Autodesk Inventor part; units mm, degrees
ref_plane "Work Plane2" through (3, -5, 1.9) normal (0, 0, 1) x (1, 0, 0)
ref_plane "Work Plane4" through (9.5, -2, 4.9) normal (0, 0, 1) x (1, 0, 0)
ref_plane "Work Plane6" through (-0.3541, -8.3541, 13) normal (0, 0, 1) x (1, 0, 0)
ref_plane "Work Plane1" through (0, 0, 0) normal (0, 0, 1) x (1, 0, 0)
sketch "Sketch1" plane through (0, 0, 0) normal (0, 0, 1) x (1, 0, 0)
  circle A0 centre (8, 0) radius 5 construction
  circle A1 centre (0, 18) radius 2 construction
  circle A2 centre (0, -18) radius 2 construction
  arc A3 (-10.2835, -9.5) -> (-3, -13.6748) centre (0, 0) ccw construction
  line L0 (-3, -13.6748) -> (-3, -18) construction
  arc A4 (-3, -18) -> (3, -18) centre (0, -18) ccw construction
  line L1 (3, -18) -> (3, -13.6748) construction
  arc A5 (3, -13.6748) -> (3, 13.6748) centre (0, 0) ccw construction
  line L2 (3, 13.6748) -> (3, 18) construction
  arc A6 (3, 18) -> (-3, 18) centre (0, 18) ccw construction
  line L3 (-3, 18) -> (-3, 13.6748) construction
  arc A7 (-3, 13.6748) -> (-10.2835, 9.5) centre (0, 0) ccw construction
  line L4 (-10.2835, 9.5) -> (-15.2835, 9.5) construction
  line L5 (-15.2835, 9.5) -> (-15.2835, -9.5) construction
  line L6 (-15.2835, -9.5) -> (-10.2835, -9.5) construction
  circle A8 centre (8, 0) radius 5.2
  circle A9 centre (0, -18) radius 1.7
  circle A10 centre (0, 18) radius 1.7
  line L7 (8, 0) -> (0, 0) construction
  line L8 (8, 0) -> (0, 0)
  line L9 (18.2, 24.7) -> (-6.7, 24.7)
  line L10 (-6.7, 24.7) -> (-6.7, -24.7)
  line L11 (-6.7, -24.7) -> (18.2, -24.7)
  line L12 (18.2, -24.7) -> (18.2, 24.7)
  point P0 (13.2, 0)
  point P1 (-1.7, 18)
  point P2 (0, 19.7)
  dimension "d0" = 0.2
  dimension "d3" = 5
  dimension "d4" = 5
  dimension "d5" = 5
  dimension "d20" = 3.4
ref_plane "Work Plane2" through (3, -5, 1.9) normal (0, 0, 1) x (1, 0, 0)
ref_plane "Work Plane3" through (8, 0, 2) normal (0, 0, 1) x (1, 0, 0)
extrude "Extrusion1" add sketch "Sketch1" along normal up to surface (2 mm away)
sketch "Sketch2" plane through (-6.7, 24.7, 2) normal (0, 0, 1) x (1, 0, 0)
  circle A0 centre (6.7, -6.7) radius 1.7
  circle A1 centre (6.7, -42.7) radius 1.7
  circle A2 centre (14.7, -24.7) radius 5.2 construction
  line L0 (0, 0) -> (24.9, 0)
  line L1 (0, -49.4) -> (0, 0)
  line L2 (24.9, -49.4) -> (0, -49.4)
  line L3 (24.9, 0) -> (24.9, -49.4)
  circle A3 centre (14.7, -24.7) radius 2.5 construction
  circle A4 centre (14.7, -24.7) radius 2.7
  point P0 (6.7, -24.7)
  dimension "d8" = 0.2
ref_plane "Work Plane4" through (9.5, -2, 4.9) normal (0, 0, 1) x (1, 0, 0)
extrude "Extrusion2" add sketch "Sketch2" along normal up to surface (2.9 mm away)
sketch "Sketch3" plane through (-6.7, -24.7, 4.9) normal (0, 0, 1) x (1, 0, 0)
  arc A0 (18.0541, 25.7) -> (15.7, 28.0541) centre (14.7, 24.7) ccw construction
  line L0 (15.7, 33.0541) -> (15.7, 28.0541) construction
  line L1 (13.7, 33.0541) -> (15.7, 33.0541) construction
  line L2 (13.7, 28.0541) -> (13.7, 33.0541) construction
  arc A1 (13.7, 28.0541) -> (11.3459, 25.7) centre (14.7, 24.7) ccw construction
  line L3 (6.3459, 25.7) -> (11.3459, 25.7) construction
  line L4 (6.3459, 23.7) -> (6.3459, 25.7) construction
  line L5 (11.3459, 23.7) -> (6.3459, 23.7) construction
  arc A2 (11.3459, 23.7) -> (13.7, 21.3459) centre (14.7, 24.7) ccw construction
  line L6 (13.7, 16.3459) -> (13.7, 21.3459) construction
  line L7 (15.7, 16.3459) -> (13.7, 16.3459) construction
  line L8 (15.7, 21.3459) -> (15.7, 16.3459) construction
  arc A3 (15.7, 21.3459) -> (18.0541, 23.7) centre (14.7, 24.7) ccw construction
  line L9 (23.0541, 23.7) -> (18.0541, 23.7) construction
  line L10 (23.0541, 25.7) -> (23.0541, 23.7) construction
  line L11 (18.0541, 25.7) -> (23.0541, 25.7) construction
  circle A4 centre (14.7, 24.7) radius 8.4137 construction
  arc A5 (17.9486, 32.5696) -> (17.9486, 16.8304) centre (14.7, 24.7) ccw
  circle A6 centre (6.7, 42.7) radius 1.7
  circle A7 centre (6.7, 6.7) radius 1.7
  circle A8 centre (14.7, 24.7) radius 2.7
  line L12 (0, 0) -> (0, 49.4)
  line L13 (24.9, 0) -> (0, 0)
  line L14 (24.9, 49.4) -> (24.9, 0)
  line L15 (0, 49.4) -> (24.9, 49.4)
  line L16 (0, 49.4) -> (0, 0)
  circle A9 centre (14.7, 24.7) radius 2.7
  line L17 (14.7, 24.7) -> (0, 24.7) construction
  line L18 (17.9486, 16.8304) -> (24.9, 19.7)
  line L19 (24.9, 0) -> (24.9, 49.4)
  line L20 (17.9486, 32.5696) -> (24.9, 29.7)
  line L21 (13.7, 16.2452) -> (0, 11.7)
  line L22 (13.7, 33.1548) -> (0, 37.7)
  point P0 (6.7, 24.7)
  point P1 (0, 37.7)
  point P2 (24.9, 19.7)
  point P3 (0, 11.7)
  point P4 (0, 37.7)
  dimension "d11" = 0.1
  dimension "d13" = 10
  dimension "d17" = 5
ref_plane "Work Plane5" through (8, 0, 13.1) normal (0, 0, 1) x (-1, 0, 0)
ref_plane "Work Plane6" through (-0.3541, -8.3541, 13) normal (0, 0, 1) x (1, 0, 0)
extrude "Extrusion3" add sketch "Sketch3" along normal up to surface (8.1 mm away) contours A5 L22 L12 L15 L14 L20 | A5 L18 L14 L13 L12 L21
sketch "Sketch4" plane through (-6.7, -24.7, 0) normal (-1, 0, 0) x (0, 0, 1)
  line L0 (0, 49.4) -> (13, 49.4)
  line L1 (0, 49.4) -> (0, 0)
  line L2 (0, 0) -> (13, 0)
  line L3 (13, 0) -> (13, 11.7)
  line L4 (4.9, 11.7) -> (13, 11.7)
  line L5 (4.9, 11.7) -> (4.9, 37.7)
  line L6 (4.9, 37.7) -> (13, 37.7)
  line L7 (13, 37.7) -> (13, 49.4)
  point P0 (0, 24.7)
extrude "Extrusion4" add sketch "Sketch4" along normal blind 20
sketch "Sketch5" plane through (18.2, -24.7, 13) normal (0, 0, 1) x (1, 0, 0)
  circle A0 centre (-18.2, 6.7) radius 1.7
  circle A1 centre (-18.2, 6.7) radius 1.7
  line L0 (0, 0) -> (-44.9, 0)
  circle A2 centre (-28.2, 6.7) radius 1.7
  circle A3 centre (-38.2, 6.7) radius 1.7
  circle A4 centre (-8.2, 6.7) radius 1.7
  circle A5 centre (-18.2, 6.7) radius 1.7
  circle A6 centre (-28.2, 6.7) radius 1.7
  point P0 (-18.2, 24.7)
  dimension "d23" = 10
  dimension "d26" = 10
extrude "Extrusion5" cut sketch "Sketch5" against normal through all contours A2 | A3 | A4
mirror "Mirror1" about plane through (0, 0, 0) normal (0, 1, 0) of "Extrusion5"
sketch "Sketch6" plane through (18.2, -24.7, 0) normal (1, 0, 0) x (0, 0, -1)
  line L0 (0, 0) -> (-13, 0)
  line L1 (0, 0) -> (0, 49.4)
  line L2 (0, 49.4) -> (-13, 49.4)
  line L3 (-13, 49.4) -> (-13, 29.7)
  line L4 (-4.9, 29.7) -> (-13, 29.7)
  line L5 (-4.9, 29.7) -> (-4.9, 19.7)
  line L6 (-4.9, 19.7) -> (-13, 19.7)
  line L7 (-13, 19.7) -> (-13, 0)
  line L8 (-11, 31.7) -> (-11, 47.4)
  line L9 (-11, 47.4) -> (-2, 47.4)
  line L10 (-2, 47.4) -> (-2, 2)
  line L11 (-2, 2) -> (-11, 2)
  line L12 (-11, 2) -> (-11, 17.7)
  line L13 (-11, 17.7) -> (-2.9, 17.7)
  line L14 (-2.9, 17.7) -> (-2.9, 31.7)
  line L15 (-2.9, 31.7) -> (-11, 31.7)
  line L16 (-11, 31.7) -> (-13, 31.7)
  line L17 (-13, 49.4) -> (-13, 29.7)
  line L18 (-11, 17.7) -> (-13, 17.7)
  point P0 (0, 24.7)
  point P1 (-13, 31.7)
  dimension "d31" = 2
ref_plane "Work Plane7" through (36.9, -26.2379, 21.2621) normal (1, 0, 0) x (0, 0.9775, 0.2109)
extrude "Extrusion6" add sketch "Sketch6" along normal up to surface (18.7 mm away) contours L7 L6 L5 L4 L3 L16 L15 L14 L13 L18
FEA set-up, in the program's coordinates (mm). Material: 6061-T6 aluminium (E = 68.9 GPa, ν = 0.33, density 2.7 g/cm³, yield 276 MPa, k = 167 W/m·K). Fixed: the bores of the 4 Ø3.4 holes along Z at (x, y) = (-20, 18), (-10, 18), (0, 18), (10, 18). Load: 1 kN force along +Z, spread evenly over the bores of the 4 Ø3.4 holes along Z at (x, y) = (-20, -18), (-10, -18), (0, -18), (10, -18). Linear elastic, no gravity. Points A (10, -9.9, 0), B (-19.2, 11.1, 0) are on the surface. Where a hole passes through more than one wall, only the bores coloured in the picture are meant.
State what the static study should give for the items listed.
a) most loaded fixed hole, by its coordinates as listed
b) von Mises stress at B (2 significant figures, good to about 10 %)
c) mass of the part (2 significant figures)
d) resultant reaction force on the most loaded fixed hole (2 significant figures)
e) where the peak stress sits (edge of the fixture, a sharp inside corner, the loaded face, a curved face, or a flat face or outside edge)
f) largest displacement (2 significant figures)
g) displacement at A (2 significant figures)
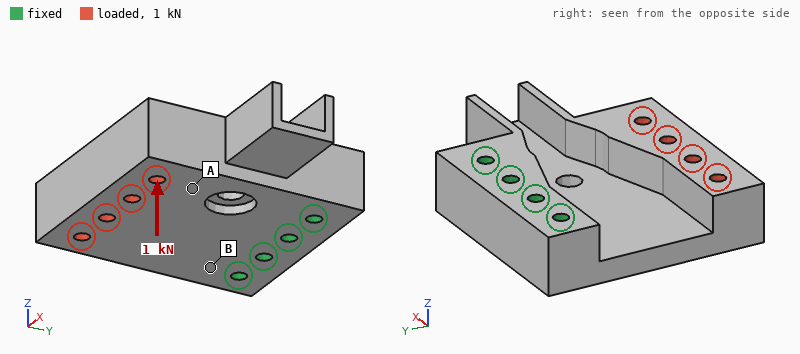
(0, 18)
130 MPa
56 g
410 N
a curved face
0.49 mm
0.19 mm
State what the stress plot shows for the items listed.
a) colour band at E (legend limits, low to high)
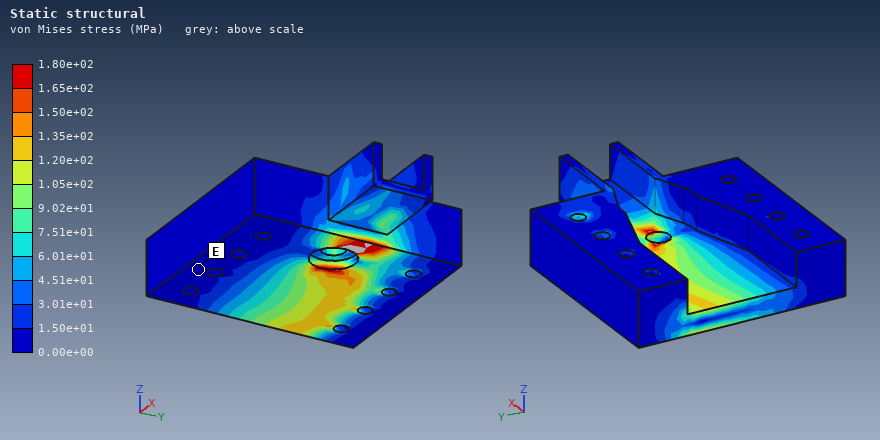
0.00e+00 to 1.50e+01 MPa
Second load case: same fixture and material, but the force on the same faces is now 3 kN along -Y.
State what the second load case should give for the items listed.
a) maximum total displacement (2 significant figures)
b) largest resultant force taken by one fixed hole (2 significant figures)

0.27 mm
1.0 kN
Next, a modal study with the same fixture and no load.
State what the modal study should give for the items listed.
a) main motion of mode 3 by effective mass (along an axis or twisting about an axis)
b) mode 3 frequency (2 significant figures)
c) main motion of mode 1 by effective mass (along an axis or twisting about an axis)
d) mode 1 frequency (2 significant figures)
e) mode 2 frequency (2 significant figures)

along X
8200 Hz
along Z
1800 Hz
4600 Hz
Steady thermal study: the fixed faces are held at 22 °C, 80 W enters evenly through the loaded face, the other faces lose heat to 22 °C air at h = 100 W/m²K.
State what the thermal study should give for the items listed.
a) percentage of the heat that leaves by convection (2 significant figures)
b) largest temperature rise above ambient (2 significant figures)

27 %
56 K
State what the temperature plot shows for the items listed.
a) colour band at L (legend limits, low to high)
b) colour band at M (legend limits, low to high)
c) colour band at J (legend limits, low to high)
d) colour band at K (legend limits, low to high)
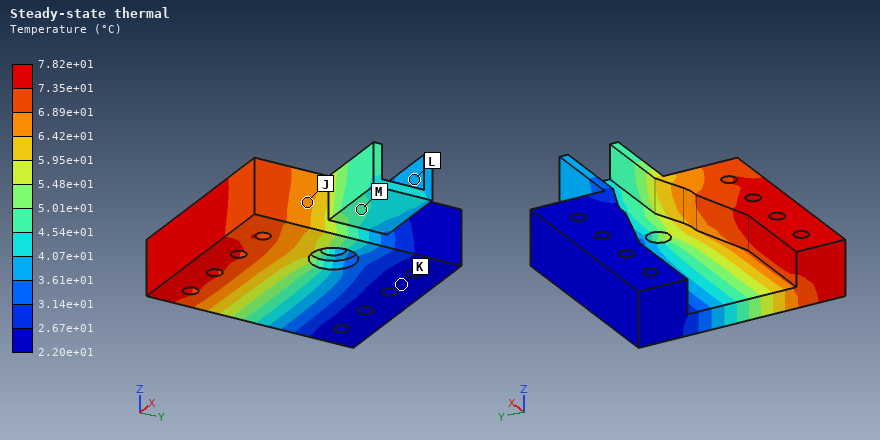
3.61e+01 to 4.07e+01 °C
4.54e+01 to 5.01e+01 °C
6.42e+01 to 6.89e+01 °C
2.20e+01 to 2.67e+01 °C
